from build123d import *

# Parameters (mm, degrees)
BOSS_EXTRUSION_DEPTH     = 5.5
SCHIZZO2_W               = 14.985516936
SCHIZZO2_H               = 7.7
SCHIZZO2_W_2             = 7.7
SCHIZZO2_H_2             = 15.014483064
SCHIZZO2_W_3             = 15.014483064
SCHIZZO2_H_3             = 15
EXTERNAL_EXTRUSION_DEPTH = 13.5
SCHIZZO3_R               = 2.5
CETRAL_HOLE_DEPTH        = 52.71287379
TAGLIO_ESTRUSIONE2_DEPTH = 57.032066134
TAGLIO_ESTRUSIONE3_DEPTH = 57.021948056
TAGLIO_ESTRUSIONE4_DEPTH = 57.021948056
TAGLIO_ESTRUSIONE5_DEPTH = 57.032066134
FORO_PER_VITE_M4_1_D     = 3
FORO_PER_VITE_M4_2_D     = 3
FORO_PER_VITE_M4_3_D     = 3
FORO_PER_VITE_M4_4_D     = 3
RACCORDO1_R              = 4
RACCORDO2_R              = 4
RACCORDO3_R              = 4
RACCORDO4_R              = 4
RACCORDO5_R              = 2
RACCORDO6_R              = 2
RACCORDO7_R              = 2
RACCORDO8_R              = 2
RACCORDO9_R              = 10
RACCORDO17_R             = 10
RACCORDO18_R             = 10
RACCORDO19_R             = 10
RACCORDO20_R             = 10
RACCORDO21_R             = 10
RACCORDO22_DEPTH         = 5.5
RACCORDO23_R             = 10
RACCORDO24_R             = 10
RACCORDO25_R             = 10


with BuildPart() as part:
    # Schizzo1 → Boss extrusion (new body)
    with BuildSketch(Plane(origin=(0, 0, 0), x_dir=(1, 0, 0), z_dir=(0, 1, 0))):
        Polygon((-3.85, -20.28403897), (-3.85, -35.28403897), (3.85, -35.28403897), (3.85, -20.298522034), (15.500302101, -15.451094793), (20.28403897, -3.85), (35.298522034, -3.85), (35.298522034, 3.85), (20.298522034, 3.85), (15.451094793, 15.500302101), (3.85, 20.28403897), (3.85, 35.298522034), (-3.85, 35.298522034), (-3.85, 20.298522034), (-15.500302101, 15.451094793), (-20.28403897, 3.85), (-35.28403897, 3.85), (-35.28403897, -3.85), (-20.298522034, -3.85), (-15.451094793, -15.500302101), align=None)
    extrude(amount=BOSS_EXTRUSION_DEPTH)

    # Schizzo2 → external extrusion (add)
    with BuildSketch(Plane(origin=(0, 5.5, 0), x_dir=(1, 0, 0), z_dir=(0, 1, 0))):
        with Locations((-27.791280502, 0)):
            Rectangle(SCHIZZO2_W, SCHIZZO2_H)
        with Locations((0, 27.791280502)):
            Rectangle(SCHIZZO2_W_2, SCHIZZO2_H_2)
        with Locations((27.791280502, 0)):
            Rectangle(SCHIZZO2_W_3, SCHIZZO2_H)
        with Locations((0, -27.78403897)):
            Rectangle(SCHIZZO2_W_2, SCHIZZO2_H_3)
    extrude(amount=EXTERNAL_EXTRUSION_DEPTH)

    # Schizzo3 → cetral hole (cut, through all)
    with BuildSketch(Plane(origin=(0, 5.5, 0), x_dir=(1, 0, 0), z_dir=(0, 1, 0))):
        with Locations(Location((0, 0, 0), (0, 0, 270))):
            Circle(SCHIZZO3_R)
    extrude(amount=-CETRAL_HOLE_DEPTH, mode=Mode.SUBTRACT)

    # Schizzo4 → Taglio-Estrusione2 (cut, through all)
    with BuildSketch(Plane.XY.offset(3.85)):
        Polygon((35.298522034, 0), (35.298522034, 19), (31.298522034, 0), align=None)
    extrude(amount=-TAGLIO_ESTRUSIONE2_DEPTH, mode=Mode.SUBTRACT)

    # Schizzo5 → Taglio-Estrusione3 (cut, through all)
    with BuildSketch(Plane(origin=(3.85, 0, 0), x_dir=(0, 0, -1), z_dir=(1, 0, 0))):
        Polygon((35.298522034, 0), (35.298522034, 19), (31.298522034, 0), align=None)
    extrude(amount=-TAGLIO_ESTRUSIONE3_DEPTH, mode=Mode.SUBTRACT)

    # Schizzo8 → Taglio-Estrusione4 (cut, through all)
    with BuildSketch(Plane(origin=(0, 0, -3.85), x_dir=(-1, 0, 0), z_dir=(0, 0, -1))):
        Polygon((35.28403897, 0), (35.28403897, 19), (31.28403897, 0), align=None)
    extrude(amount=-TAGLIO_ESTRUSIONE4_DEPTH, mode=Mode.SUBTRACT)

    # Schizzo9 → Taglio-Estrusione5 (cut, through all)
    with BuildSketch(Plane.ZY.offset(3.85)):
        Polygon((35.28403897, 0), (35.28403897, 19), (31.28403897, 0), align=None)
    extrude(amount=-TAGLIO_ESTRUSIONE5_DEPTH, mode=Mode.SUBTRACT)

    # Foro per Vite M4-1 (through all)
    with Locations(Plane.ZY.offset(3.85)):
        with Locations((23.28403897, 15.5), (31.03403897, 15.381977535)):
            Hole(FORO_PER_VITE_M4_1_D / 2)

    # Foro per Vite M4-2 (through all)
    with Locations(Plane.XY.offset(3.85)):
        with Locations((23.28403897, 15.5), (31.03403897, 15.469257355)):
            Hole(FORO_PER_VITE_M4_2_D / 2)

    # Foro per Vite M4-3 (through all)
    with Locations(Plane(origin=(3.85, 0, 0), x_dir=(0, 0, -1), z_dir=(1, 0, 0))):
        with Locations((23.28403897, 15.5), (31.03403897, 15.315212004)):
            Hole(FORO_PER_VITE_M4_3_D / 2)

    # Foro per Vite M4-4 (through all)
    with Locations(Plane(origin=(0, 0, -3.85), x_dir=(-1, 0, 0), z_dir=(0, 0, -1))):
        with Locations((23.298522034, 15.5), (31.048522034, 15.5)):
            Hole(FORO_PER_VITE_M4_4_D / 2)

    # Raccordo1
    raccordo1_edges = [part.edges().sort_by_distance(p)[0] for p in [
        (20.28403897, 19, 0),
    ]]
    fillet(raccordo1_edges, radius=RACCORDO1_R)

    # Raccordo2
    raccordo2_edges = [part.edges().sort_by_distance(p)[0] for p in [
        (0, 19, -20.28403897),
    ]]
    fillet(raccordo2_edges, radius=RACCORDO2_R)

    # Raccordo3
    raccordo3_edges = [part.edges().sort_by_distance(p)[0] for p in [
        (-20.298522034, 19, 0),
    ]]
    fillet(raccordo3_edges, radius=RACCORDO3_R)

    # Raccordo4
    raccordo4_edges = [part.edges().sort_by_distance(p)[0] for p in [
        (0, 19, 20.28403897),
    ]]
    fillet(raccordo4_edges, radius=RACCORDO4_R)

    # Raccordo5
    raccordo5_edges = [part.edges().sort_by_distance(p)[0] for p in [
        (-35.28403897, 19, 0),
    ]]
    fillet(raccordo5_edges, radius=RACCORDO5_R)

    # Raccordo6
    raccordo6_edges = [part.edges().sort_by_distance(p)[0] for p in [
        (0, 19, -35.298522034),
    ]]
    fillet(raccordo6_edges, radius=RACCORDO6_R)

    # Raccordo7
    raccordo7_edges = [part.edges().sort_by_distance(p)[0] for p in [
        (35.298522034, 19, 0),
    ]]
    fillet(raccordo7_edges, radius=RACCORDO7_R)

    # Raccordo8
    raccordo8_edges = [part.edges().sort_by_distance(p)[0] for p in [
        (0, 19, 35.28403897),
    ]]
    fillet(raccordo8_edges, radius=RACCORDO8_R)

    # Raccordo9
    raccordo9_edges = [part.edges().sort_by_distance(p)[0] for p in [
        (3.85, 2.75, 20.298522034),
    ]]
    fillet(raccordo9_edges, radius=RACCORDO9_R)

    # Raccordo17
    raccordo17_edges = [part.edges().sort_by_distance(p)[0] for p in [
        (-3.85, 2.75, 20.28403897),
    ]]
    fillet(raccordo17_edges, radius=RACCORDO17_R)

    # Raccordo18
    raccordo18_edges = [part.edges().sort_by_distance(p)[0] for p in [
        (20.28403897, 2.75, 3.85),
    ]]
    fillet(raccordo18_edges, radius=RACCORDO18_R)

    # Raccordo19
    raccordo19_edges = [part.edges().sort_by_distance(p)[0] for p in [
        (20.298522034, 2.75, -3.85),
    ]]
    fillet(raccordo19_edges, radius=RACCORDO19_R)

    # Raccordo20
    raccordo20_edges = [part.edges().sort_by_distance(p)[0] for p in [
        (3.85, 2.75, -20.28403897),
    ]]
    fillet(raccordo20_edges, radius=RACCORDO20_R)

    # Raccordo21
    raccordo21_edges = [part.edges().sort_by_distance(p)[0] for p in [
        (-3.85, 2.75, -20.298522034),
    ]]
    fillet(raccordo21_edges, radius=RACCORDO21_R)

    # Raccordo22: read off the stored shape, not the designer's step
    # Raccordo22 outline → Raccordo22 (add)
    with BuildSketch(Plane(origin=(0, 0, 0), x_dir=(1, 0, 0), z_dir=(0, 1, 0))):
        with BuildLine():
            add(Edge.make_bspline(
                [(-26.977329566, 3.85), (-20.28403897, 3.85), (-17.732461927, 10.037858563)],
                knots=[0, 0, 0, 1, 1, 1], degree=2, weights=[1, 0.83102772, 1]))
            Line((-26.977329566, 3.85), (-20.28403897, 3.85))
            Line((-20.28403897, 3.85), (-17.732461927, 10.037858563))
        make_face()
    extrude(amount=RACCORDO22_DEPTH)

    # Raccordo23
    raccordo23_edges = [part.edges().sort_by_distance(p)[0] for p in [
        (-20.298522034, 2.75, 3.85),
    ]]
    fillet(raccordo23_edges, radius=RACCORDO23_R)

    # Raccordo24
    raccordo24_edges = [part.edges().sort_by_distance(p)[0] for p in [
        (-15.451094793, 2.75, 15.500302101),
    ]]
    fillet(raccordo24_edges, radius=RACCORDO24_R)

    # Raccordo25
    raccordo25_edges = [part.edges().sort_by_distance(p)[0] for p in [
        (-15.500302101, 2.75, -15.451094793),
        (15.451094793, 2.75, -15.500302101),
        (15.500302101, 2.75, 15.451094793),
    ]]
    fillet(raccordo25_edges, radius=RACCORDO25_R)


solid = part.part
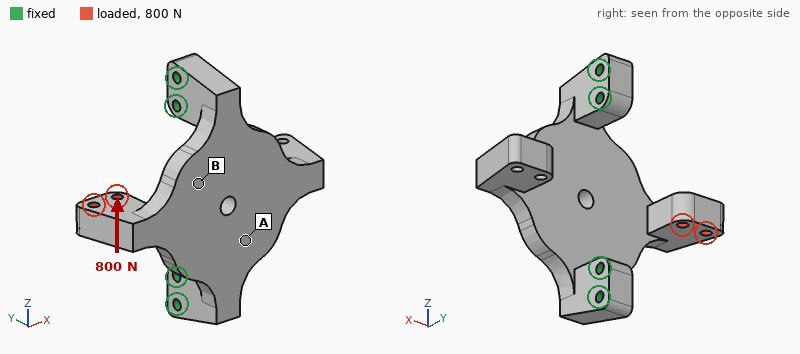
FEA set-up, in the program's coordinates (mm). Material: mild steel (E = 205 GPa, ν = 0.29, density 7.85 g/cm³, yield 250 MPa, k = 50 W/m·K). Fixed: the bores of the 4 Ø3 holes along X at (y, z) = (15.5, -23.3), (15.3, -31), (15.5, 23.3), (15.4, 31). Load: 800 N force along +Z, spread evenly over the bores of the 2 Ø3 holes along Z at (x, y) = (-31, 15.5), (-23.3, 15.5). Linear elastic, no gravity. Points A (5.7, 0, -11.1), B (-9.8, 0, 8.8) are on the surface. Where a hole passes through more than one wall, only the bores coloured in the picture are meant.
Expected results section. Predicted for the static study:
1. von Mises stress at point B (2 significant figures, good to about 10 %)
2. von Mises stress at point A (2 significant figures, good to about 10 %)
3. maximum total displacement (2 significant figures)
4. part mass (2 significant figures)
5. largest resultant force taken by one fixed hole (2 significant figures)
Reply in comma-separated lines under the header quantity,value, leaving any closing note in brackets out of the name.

quantity,value
von Mises stress at point B,42 MPa
von Mises stress at point A,20 MPa
maximum total displacement,66 µm
part mass,110 g
largest resultant force taken by one fixed hole,820 N
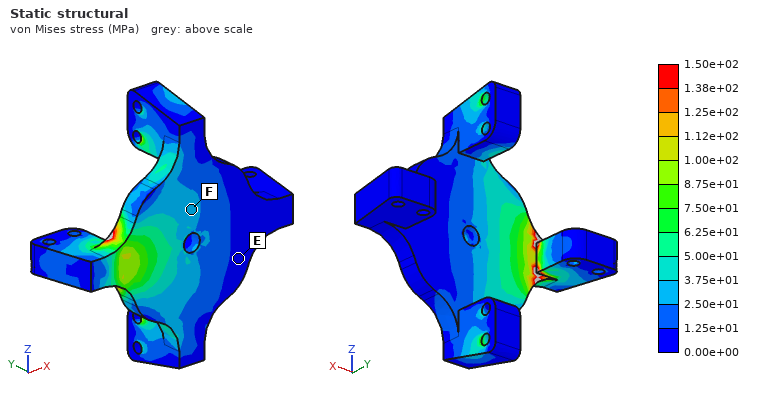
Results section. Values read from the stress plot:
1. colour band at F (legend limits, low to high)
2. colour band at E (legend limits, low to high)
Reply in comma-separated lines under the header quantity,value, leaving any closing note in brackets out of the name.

quantity,value
colour band at F,2.50e+01 to 3.75e+01 MPa
colour band at E,0.00e+00 to 1.25e+01 MPa
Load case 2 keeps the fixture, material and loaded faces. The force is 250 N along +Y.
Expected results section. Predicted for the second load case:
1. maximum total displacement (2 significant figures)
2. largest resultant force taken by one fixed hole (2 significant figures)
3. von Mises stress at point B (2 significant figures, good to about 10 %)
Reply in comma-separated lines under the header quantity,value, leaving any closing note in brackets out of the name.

quantity,value
maximum total displacement,72 µm
largest resultant force taken by one fixed hole,130 N
von Mises stress at point B,32 MPa
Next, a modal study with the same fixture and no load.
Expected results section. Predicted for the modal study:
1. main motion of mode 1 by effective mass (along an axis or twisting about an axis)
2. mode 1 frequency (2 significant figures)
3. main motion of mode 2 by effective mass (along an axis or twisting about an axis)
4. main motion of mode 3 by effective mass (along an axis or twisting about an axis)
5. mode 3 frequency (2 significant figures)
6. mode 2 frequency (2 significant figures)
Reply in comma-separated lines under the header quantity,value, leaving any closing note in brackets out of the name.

quantity,value
main motion of mode 1 by effective mass,twisting about Z
mode 1 frequency,2200 Hz
main motion of mode 2 by effective mass,along Y
main motion of mode 3 by effective mass,twisting about Y
mode 3 frequency,6600 Hz
mode 2 frequency,3500 Hz
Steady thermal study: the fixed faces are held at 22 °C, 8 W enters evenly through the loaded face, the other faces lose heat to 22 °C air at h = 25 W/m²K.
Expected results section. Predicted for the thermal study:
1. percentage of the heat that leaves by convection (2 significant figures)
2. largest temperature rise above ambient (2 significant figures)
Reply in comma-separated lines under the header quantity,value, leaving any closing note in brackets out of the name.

quantity,value
percentage of the heat that leaves by convection,35 %
largest temperature rise above ambient,62 K
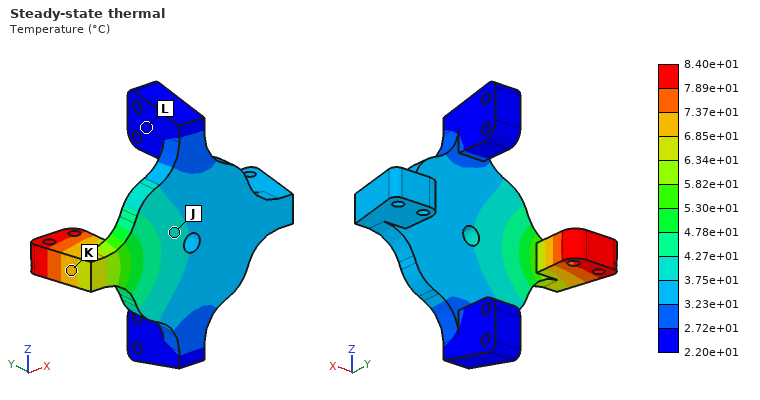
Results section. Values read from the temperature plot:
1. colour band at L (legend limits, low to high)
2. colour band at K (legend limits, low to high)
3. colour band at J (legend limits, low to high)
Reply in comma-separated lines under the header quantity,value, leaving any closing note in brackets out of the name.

quantity,value
colour band at L,2.20e+01 to 2.72e+01 °C
colour band at K,6.85e+01 to 7.37e+01 °C
colour band at J,3.75e+01 to 4.27e+01 °C
